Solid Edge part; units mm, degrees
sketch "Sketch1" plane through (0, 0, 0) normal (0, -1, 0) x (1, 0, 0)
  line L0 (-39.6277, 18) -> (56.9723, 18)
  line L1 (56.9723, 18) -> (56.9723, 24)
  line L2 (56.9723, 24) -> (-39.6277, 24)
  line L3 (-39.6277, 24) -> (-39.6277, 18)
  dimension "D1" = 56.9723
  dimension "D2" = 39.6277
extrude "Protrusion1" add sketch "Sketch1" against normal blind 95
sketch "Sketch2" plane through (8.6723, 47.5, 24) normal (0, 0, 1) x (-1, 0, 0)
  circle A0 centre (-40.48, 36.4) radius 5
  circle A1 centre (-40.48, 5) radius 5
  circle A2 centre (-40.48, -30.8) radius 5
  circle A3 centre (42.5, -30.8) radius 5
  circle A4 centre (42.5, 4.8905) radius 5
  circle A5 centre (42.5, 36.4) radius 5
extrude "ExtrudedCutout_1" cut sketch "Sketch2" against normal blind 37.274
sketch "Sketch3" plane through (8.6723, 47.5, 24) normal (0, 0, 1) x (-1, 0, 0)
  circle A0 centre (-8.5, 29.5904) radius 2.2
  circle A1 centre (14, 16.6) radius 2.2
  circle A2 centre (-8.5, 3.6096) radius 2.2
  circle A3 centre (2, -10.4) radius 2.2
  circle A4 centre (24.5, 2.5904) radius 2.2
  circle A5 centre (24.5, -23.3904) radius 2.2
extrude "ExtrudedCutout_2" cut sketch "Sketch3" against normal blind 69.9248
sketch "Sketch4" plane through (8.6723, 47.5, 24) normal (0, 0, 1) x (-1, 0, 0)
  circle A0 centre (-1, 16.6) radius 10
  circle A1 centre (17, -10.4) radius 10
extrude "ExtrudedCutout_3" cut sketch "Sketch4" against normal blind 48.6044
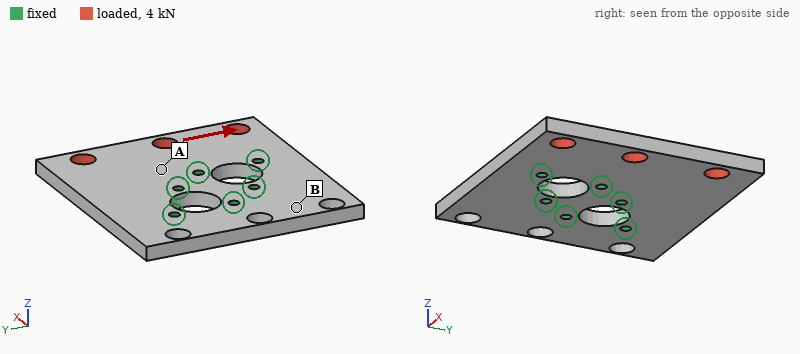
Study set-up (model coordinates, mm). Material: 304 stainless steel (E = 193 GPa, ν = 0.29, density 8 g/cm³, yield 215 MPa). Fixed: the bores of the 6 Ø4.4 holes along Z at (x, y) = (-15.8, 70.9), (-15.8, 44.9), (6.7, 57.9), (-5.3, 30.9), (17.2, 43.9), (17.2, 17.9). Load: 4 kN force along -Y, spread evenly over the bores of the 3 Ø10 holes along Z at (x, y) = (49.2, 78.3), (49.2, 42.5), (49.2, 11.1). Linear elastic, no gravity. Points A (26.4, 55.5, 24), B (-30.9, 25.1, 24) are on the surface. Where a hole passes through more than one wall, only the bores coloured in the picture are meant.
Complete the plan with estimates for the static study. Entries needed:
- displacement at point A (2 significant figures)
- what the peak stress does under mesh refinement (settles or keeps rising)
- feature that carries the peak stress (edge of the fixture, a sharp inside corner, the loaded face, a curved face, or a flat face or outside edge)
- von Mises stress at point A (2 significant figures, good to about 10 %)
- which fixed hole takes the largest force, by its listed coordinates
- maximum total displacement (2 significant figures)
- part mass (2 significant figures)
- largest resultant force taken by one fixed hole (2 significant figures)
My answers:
2.5 µm
keeps rising
edge of the fixture
17 MPa
(17.2, 17.9)
10 µm
380 g
2.6 kN
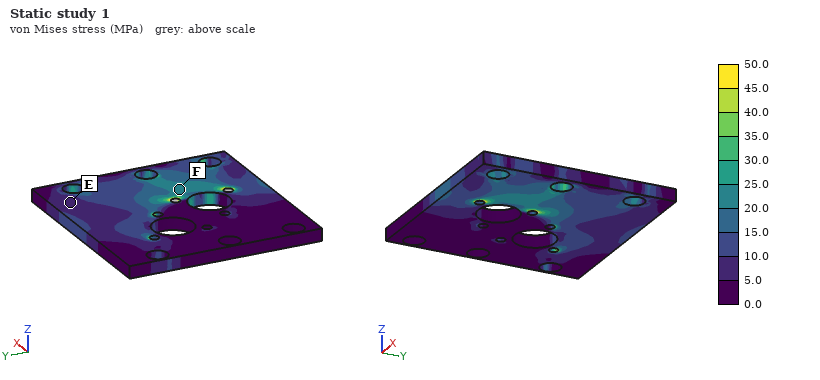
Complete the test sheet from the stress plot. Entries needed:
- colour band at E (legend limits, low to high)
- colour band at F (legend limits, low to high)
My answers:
5.0 to 10.0 MPa
20.0 to 25.0 MPa
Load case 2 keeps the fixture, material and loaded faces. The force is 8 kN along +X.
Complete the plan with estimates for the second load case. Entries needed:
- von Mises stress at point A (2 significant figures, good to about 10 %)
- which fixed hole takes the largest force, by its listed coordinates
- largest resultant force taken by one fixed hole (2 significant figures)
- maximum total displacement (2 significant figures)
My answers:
15 MPa
(17.2, 17.9)
2.6 kN
7.5 µm
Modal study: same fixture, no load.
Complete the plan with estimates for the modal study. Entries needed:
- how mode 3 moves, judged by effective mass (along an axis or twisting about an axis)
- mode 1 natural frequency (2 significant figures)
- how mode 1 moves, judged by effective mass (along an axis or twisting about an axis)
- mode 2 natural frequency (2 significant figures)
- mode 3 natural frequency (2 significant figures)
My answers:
along Z
2000 Hz
along Z
3200 Hz
3800 Hz
